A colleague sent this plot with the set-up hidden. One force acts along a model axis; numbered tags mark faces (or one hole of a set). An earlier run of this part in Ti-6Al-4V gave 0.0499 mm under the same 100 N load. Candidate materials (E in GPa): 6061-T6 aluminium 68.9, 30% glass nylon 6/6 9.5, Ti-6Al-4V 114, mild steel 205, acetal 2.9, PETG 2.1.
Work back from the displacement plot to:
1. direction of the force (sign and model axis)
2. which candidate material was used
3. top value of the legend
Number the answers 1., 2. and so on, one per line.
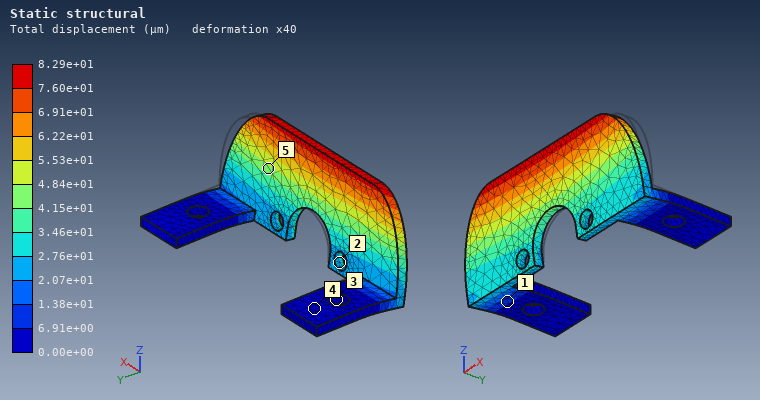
1. -Z
2. 6061-T6 aluminium
3. 8.29e+01 µm
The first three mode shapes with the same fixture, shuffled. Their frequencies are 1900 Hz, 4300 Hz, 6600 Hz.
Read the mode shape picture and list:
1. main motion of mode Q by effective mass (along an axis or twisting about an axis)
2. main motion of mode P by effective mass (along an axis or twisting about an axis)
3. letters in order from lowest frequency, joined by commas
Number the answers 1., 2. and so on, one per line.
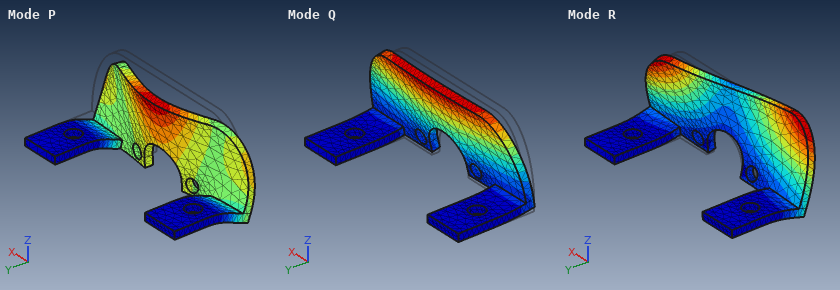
1. along Y
2. along Z
3. Q, R, P
